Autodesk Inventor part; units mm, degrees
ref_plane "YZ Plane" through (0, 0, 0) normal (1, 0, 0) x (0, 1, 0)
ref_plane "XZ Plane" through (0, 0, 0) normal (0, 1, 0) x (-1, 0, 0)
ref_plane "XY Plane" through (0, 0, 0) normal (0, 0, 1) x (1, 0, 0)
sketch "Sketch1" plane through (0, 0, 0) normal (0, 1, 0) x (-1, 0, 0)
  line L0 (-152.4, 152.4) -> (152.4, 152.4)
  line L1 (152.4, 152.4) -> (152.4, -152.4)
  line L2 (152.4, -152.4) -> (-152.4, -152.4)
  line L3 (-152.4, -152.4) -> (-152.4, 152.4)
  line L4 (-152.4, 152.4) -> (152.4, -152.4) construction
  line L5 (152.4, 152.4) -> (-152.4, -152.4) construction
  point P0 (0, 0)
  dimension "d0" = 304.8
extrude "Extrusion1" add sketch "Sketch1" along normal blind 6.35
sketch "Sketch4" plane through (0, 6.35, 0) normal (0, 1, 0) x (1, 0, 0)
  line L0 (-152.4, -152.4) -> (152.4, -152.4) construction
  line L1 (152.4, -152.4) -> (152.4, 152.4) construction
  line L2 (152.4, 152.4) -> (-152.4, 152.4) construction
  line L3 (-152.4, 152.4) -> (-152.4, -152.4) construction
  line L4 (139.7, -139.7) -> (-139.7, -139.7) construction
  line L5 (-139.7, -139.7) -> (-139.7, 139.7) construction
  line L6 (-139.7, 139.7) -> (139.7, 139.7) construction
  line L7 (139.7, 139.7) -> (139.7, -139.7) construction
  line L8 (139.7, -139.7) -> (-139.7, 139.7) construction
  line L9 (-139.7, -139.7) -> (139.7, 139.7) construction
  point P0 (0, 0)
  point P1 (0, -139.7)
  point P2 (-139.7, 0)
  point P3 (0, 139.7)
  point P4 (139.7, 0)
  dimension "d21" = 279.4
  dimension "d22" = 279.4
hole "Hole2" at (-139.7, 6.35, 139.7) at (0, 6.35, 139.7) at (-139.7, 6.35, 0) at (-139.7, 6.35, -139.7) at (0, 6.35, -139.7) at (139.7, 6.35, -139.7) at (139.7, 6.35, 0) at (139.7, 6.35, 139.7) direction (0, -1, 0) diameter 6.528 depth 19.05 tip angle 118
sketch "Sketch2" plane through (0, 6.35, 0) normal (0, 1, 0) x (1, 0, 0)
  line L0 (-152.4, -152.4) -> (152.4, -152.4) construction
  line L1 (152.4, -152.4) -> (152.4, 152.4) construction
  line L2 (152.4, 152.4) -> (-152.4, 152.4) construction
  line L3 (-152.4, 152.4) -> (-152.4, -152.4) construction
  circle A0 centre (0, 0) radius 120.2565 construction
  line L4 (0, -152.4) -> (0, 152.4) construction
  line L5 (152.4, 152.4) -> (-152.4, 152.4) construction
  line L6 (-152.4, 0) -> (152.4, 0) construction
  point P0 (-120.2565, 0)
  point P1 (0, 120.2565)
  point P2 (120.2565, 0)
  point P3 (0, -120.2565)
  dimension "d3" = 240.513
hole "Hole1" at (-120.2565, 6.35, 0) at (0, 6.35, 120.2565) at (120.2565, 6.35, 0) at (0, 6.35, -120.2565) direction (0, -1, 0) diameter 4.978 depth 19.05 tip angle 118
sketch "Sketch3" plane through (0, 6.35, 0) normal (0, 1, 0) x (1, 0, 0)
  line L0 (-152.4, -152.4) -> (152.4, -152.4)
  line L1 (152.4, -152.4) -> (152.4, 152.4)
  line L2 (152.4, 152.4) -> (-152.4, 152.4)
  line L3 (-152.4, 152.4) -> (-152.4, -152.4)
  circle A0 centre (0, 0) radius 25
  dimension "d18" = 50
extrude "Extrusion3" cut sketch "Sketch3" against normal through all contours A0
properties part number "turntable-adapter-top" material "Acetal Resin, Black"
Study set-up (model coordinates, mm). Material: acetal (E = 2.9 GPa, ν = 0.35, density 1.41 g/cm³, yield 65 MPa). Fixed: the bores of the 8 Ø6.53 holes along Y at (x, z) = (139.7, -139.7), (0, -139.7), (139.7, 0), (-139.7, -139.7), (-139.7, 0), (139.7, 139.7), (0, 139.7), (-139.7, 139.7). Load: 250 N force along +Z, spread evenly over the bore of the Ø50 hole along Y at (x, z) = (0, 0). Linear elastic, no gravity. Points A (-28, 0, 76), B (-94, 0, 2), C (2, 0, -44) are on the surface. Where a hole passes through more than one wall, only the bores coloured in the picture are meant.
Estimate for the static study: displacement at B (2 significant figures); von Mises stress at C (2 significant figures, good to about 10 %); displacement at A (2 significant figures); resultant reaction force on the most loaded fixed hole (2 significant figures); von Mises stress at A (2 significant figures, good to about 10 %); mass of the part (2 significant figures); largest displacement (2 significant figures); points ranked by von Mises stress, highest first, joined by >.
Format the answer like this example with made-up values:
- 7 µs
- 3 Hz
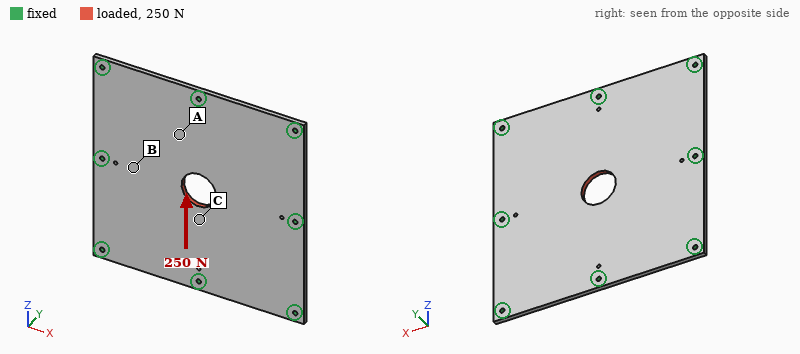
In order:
- 2.7 µm
- 0.23 MPa
- 4.8 µm
- 57 N
- 0.13 MPa
- 810 g
- 8.8 µm
- C > A > B
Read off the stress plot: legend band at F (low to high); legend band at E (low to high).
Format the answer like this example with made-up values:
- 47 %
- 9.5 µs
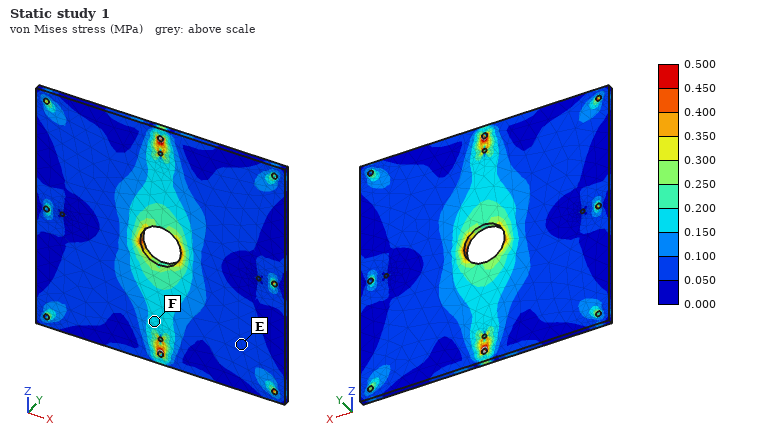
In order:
- 0.150 to 0.200 MPa
- 0.050 to 0.100 MPa
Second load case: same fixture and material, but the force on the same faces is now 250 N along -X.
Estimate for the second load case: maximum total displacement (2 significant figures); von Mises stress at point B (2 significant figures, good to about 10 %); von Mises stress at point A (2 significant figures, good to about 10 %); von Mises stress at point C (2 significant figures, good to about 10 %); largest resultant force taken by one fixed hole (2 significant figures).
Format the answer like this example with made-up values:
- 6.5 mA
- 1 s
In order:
- 8.8 µm
- 0.17 MPa
- 0.063 MPa
- 0.12 MPa
- 57 N
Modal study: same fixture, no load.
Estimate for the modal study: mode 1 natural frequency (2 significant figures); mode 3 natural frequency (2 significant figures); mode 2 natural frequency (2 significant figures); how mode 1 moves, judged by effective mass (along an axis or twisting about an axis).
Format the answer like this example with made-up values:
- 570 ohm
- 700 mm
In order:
- 160 Hz
- 290 Hz
- 290 Hz
- along Y
